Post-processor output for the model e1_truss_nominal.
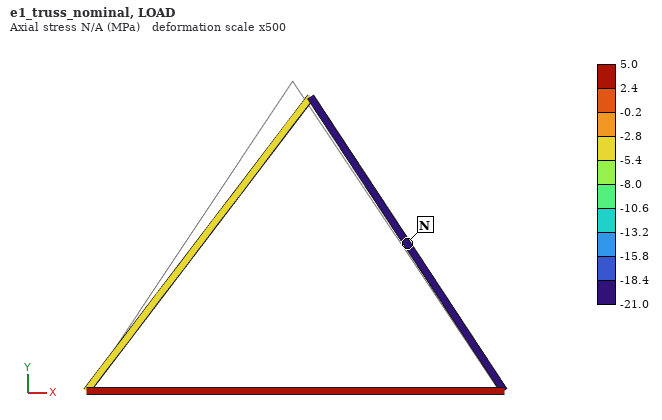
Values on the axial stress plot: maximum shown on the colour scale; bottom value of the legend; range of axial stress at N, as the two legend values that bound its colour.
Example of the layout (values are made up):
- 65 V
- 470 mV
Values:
- 5.0 MPa
- -21.0 MPa
- -21.0 to -18.4 MPa
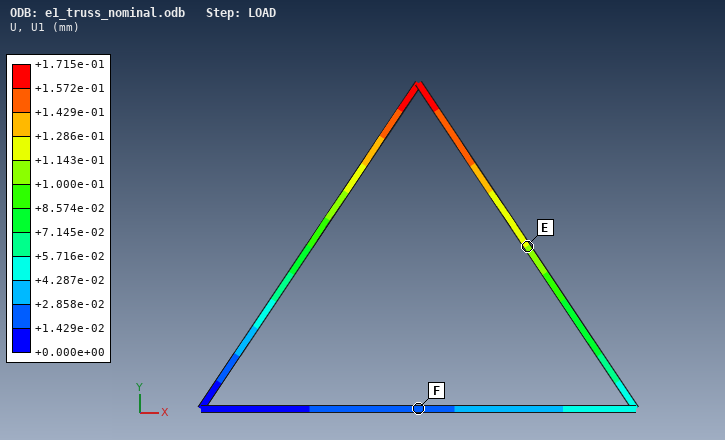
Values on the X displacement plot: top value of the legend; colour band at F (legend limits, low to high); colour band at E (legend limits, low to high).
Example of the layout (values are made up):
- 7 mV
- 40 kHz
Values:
- +1.715e-01 mm
- +1.429e-02 to +2.858e-02 mm
- +1.000e-01 to +1.143e-01 mm
